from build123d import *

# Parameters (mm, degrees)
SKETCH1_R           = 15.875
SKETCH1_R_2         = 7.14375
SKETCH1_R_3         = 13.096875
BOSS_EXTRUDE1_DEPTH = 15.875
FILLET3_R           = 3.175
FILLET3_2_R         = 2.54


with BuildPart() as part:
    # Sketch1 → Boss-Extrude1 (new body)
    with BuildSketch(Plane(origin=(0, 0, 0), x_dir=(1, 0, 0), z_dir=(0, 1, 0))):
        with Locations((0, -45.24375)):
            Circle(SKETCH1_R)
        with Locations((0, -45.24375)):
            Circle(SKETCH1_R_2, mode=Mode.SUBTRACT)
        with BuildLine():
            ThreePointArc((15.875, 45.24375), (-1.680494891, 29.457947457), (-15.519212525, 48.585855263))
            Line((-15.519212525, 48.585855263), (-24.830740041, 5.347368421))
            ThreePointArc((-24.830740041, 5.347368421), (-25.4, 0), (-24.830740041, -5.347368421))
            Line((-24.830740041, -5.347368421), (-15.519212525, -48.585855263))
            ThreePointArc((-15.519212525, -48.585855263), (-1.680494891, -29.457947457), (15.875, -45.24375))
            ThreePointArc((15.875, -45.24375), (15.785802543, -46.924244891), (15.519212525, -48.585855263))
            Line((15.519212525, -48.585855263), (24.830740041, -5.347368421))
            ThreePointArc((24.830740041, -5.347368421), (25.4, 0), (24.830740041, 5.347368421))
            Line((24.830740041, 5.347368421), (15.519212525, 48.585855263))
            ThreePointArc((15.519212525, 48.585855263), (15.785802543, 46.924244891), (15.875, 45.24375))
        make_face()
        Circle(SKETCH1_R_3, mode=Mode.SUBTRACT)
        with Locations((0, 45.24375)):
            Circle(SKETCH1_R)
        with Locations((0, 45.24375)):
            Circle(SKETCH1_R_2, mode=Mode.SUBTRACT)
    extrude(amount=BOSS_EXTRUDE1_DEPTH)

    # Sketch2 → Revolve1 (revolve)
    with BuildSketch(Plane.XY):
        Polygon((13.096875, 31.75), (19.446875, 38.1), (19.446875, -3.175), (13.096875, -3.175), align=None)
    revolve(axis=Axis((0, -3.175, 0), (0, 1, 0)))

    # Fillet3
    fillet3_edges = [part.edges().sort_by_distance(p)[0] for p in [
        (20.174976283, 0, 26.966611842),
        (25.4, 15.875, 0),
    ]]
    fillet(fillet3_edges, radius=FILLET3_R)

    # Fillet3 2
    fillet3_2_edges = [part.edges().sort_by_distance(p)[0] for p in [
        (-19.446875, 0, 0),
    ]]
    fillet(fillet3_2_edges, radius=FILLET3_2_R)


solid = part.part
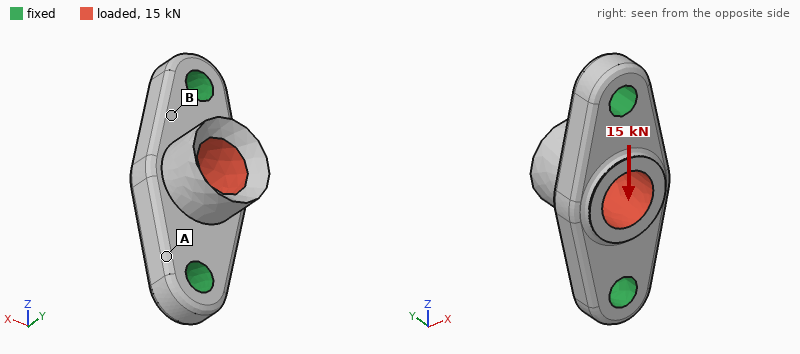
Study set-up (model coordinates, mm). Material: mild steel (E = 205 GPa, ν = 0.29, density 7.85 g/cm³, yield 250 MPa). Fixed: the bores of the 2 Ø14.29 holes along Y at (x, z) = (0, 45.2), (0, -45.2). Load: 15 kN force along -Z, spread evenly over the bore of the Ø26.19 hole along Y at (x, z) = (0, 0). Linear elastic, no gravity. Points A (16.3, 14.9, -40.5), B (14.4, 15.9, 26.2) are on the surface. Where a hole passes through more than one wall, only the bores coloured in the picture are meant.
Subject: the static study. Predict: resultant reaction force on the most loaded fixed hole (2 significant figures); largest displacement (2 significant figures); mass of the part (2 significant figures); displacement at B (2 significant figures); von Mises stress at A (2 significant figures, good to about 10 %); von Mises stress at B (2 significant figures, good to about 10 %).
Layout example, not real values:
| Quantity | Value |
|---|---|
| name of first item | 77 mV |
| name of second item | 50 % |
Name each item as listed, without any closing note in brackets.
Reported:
| Quantity | Value |
|---|---|
| resultant reaction force on the most loaded fixed hole | 7.6 kN |
| largest displacement | 7.3 µm |
| mass of the part | 570 g |
| displacement at B | 1.5 µm |
| von Mises stress at A | 5.5 MPa |
| von Mises stress at B | 15 MPa |
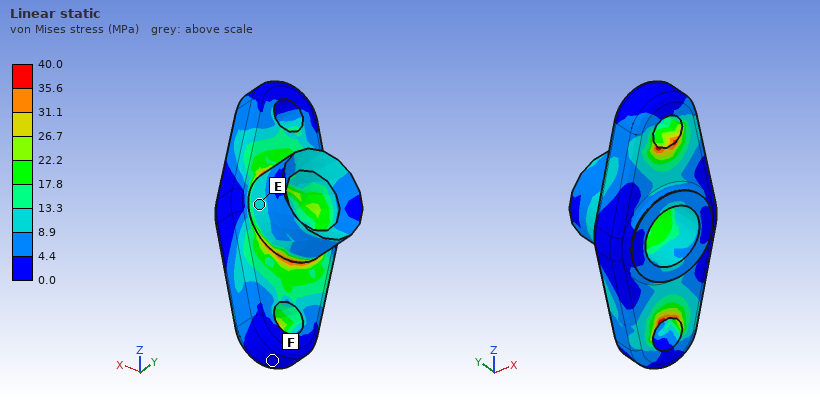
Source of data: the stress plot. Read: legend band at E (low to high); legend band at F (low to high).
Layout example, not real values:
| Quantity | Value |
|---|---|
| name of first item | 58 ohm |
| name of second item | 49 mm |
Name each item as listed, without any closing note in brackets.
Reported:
| Quantity | Value |
|---|---|
| legend band at E | 8.9 to 13.3 MPa |
| legend band at F | 0.0 to 4.4 MPa |
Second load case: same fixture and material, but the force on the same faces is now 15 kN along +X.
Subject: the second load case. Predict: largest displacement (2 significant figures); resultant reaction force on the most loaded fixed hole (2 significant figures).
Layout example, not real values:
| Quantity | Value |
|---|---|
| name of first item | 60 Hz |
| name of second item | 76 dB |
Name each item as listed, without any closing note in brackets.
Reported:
| Quantity | Value |
|---|---|
| largest displacement | 24 µm |
| resultant reaction force on the most loaded fixed hole | 7.5 kN |
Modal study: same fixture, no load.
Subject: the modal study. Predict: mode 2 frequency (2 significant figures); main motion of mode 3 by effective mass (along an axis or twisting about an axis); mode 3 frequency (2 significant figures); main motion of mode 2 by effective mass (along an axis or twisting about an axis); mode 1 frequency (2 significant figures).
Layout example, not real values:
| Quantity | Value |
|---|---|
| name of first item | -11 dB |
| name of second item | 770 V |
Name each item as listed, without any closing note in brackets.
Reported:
| Quantity | Value |
|---|---|
| mode 2 frequency | 8600 Hz |
| main motion of mode 3 by effective mass | along X |
| mode 3 frequency | 13 kHz |
| main motion of mode 2 by effective mass | along Y |
| mode 1 frequency | 7500 Hz |
